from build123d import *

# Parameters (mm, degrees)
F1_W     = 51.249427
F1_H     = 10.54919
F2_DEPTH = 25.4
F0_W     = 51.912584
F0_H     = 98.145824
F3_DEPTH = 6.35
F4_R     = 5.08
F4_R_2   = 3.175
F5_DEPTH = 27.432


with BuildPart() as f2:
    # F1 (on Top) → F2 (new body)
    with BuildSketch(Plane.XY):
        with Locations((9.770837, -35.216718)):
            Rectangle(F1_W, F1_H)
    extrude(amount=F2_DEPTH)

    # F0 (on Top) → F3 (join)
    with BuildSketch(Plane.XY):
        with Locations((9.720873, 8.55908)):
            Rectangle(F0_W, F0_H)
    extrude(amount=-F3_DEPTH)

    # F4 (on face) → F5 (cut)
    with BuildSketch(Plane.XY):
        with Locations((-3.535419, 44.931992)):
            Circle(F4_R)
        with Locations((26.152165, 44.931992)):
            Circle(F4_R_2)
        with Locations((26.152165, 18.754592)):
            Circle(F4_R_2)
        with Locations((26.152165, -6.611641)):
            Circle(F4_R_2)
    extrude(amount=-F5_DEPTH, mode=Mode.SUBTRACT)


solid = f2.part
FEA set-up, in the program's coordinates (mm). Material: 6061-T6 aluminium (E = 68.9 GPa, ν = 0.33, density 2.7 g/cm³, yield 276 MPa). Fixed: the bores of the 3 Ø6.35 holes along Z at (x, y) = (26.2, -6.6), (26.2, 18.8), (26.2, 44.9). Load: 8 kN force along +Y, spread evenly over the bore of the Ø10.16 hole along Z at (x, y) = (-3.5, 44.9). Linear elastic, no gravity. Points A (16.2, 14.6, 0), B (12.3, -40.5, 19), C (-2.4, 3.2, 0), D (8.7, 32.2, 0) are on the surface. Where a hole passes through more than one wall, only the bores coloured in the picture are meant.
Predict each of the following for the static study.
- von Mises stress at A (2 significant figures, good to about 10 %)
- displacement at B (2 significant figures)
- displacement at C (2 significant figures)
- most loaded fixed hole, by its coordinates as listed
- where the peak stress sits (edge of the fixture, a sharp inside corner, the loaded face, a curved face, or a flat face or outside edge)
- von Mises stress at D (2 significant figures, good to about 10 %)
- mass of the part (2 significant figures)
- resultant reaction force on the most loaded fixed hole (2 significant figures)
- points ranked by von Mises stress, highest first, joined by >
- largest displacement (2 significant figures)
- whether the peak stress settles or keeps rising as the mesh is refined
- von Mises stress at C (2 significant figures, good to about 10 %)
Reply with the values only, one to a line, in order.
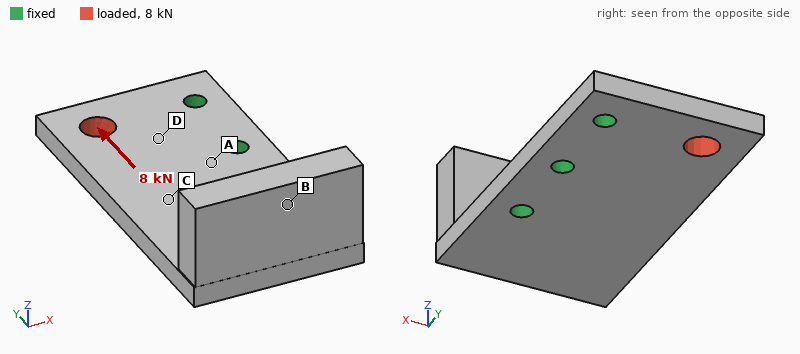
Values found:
34 MPa
27 µm
22 µm
(26.2, 44.9)
edge of the fixture
47 MPa
120 g
5.2 kN
D > A > C > B
52 µm
keeps rising
20 MPa
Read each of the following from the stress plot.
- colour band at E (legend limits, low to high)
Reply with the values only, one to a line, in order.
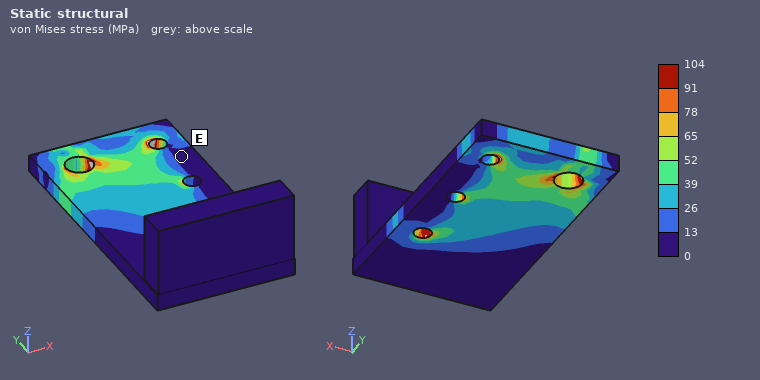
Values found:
0 to 13 MPa
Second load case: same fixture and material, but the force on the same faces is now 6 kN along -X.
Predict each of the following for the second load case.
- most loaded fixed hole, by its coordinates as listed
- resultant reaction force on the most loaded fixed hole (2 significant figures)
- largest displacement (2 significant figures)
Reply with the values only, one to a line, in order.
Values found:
(26.2, 44.9)
5.1 kN
27 µm
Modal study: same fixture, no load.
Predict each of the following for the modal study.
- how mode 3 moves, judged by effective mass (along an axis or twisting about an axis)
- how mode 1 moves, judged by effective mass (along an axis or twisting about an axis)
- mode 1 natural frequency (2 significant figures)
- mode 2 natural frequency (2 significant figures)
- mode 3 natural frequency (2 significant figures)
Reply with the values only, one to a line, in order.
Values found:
along Z
along Z
1300 Hz
2100 Hz
3700 Hz
